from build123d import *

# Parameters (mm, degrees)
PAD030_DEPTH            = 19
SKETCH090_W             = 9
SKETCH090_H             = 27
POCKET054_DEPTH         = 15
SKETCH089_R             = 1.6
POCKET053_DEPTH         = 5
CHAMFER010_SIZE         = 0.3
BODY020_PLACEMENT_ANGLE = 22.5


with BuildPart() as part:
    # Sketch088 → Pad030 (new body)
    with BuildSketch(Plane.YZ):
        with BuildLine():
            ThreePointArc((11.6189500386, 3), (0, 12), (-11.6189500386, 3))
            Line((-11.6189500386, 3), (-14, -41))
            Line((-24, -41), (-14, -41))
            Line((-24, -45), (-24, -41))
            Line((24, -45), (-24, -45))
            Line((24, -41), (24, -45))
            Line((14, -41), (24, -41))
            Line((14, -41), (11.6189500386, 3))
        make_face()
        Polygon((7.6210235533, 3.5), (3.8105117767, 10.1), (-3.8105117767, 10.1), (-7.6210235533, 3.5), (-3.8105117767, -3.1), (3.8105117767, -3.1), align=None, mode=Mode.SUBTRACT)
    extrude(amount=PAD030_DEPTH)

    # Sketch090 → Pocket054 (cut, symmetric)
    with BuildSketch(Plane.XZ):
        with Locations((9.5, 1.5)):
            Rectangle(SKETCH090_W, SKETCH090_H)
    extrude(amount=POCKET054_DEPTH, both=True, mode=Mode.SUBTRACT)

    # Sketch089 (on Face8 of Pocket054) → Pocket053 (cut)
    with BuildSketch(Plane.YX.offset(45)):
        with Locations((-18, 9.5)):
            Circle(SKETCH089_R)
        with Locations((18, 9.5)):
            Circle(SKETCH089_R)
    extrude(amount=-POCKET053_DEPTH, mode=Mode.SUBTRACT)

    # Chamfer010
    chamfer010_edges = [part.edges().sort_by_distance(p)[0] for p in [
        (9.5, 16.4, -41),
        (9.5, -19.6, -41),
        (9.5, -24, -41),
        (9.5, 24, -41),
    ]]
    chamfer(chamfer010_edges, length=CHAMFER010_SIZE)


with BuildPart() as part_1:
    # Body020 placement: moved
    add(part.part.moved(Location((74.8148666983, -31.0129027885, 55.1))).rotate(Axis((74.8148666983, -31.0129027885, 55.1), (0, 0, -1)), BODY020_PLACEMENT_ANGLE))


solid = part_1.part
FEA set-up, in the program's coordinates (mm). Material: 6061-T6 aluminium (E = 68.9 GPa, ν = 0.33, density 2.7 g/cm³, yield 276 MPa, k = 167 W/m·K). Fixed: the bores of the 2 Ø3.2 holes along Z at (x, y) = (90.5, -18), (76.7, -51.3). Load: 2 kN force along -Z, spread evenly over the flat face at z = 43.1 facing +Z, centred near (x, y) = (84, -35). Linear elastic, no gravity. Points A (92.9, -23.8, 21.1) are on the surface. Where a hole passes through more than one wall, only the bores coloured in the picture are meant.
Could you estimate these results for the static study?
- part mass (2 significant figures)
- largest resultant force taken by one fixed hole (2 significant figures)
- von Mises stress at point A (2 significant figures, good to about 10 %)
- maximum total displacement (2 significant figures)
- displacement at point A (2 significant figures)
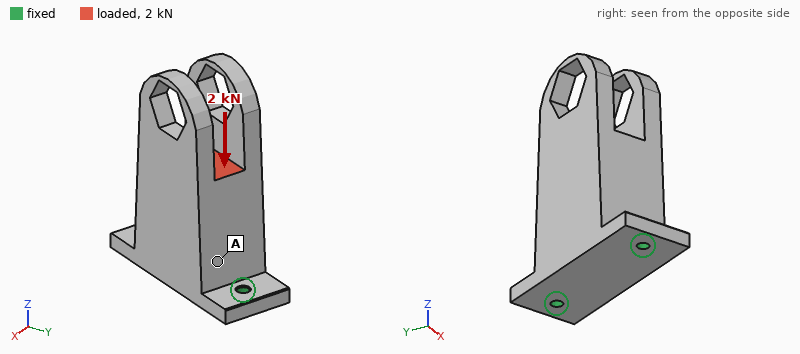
59 g
1.1 kN
11 MPa
12 µm
9.3 µm
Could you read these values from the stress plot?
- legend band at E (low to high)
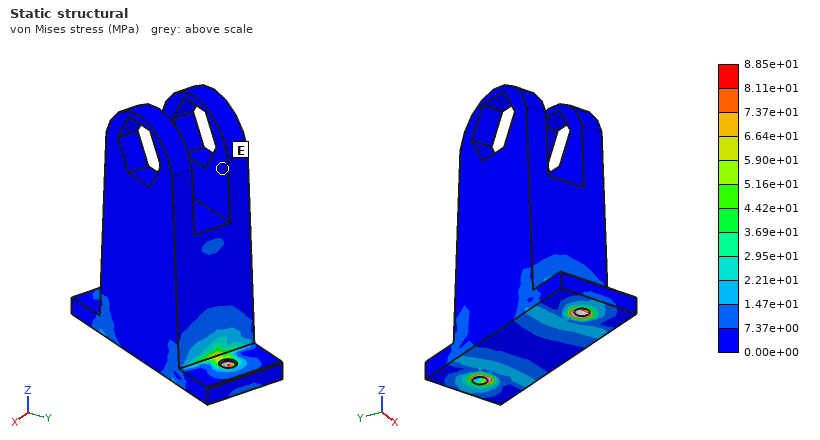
0.00e+00 to 7.37e+00 MPa
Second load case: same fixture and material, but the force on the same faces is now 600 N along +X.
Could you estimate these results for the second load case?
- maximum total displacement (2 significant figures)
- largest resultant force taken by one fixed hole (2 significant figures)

0.28 mm
380 N
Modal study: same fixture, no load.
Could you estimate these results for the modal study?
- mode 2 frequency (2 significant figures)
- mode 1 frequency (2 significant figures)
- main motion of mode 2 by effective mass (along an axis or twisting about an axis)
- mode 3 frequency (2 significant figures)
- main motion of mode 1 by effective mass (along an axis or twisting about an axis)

5800 Hz
1700 Hz
along Y
8700 Hz
along X
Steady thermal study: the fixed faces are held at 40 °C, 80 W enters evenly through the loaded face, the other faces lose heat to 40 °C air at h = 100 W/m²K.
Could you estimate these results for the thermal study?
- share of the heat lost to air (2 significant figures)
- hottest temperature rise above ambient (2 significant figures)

26 %
48 K
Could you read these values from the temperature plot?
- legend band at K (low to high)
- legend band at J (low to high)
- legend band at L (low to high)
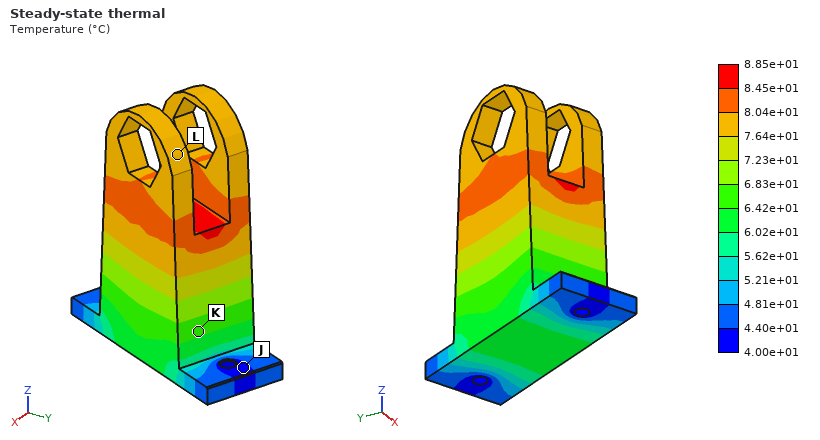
6.42e+01 to 6.83e+01 °C
4.00e+01 to 4.40e+01 °C
7.64e+01 to 8.04e+01 °C
